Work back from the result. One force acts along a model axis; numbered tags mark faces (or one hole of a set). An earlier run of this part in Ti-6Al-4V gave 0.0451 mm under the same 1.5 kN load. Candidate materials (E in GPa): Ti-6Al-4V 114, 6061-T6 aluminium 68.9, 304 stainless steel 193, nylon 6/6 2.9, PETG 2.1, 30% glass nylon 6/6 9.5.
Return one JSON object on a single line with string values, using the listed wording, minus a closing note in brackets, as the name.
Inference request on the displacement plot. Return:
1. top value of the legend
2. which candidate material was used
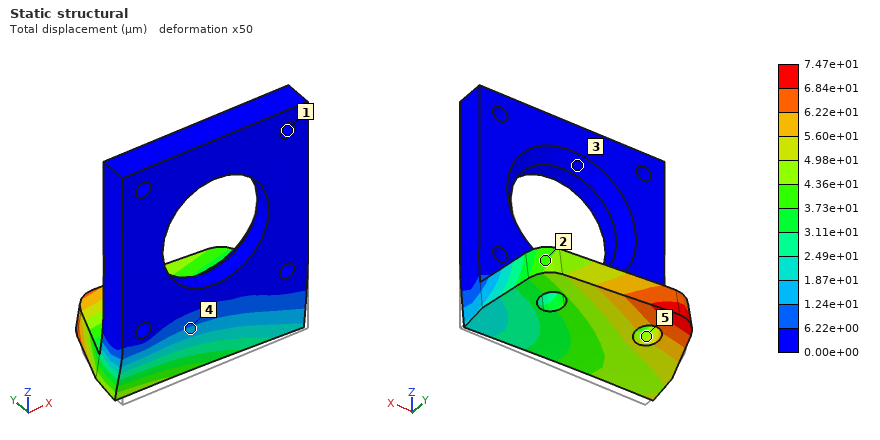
{"top value of the legend": "7.47e+01 µm", "which candidate material was used": "6061-T6 aluminium"}
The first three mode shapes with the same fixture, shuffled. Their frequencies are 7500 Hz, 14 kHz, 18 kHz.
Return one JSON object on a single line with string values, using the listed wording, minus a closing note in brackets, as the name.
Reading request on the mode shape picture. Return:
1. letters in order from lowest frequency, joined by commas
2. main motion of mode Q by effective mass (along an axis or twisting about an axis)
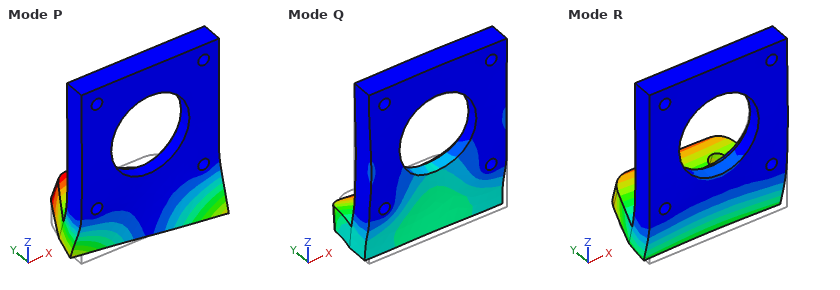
{"letters in order from lowest frequency, joined by commas": "R, P, Q", "main motion of mode Q by effective mass": "along Y"}
